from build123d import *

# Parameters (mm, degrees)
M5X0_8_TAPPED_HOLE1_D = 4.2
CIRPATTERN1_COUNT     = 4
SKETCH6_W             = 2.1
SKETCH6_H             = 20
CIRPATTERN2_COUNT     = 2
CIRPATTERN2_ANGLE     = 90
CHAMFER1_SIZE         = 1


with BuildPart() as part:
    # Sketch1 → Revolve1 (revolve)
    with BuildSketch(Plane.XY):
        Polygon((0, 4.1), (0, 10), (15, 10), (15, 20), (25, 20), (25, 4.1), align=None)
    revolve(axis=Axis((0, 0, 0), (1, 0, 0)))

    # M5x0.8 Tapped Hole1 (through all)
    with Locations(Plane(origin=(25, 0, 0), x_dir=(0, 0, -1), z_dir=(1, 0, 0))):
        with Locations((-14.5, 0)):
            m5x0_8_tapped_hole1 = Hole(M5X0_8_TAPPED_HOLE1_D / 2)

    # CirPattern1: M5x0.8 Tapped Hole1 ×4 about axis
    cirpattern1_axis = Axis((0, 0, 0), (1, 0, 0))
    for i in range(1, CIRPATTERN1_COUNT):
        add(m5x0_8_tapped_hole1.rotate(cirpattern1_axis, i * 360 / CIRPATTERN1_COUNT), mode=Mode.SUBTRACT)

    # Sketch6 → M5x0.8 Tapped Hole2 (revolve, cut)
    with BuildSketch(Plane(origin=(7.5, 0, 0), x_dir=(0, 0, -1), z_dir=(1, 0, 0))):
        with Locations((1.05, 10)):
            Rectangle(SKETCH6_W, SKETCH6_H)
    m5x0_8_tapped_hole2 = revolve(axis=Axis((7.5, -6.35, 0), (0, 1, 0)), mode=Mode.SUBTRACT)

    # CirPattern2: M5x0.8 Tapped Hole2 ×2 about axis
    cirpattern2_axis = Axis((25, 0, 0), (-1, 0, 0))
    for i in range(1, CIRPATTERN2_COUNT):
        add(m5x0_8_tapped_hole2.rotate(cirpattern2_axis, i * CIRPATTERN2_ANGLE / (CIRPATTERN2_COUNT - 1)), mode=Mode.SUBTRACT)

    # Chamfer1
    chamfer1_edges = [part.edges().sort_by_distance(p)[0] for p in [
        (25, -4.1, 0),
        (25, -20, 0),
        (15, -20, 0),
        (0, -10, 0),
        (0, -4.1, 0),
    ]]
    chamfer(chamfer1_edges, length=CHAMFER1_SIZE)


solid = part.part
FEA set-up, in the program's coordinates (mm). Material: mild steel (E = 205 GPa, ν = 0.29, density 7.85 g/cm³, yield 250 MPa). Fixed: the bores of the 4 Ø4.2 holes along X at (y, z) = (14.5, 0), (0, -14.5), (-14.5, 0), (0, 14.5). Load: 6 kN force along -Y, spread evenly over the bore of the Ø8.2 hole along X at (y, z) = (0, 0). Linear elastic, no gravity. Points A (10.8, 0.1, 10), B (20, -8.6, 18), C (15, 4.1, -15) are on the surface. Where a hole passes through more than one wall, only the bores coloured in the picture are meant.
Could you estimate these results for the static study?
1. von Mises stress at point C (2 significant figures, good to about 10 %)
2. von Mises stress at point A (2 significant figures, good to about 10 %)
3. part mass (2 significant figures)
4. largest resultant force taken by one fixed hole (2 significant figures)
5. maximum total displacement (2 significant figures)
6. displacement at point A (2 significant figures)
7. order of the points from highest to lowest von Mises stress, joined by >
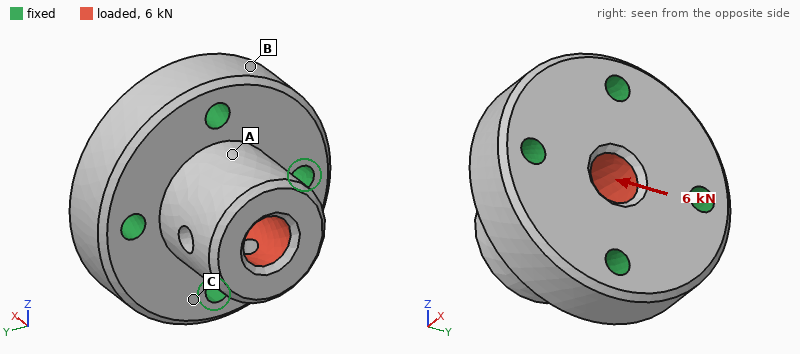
10 MPa
18 MPa
120 g
2.4 kN
5.7 µm
2.1 µm
A > C > B
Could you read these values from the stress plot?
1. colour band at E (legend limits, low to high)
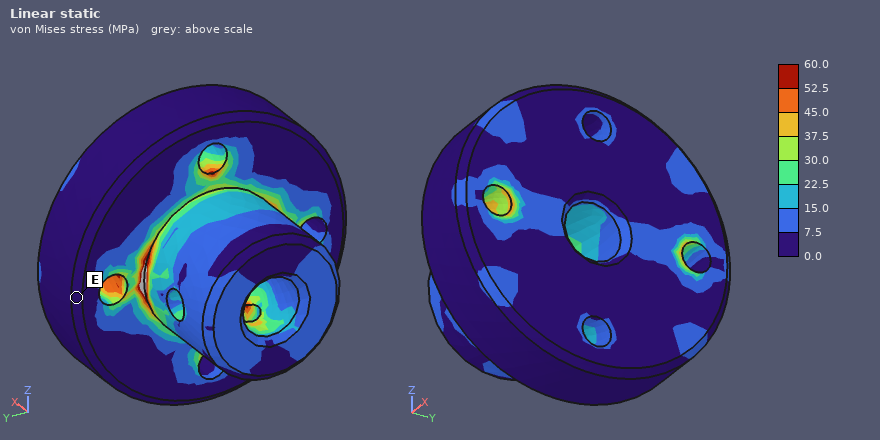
0.0 to 7.5 MPa
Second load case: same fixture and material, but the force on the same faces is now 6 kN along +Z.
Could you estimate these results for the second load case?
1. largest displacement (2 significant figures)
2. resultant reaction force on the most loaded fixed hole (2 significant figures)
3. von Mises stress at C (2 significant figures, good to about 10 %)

5.7 µm
2.4 kN
12 MPa
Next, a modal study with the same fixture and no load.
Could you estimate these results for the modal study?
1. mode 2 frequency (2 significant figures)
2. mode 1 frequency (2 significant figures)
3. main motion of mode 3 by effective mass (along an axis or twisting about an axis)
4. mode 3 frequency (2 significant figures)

27 kHz
27 kHz
along X
43 kHz
